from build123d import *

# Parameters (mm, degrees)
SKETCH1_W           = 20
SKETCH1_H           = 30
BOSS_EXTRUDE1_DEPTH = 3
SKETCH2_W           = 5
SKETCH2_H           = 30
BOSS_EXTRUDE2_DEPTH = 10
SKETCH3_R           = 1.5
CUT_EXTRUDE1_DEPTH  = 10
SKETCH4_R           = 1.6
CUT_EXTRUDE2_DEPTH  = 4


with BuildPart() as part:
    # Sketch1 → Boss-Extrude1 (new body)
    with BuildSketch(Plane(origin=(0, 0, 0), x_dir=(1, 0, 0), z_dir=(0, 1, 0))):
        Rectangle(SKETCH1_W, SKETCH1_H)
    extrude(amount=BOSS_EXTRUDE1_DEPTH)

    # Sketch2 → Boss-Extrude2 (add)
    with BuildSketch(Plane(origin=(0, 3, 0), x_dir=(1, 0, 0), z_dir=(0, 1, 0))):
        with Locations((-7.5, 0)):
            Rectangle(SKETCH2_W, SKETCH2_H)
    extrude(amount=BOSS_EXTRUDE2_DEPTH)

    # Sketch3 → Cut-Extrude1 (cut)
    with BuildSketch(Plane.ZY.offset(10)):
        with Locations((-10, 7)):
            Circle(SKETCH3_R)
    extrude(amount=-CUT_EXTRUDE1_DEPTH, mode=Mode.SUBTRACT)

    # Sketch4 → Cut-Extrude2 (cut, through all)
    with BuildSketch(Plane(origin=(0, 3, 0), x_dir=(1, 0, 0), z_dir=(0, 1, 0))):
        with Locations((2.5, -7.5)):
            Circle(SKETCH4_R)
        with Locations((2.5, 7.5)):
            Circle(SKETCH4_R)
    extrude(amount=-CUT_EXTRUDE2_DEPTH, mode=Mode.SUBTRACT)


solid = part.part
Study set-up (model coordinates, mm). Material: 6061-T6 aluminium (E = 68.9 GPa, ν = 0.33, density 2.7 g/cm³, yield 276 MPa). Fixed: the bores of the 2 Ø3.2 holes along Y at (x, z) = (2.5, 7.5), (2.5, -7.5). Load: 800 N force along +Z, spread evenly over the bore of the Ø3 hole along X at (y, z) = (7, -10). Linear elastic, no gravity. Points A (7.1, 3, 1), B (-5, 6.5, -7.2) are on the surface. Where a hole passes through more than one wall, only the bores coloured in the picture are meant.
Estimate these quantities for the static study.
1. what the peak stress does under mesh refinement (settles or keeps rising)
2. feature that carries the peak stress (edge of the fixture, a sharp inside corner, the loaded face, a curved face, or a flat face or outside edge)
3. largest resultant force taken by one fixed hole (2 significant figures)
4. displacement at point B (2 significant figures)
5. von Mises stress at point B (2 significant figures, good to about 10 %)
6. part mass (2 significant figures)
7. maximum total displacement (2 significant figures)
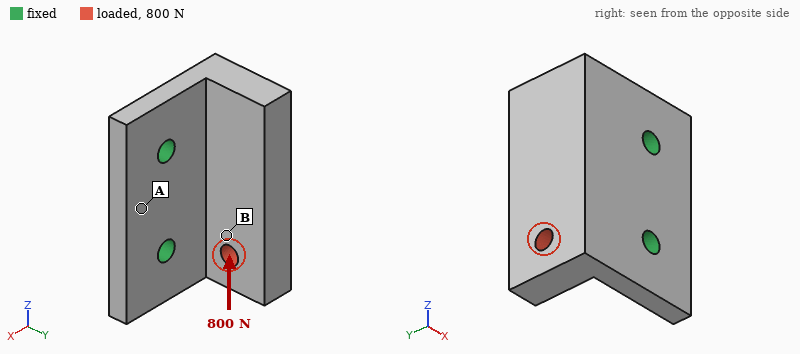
keeps rising
edge of the fixture
650 N
16 µm
28 MPa
8.7 g
31 µm
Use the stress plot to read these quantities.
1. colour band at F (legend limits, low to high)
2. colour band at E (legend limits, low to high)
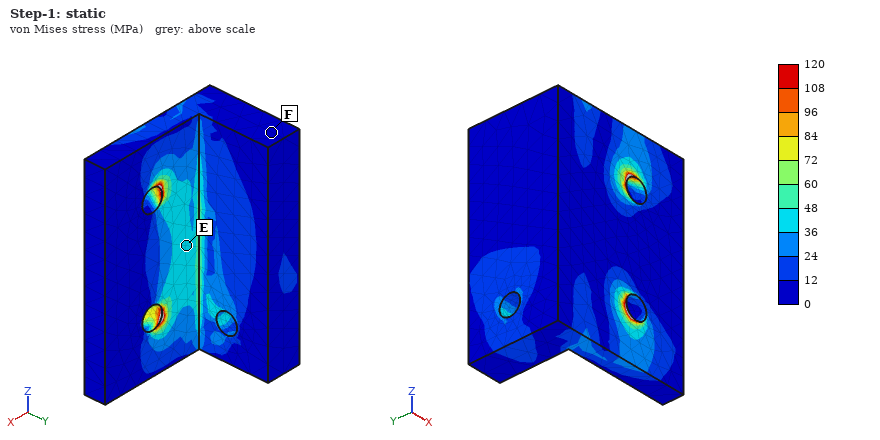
0 to 12 MPa
36 to 48 MPa
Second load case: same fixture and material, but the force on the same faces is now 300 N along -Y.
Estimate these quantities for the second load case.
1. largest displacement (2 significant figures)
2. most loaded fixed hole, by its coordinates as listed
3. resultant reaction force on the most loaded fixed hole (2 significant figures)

62 µm
(2.5, -7.5)
310 N
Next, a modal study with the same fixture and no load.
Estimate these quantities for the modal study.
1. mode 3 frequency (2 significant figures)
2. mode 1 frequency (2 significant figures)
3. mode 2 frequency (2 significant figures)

20 kHz
5900 Hz
11 kHz
